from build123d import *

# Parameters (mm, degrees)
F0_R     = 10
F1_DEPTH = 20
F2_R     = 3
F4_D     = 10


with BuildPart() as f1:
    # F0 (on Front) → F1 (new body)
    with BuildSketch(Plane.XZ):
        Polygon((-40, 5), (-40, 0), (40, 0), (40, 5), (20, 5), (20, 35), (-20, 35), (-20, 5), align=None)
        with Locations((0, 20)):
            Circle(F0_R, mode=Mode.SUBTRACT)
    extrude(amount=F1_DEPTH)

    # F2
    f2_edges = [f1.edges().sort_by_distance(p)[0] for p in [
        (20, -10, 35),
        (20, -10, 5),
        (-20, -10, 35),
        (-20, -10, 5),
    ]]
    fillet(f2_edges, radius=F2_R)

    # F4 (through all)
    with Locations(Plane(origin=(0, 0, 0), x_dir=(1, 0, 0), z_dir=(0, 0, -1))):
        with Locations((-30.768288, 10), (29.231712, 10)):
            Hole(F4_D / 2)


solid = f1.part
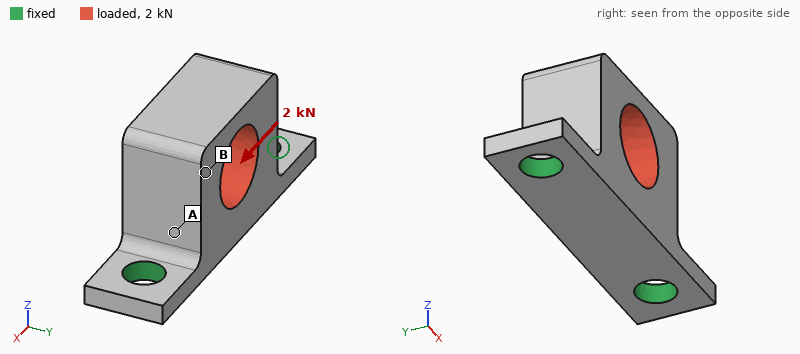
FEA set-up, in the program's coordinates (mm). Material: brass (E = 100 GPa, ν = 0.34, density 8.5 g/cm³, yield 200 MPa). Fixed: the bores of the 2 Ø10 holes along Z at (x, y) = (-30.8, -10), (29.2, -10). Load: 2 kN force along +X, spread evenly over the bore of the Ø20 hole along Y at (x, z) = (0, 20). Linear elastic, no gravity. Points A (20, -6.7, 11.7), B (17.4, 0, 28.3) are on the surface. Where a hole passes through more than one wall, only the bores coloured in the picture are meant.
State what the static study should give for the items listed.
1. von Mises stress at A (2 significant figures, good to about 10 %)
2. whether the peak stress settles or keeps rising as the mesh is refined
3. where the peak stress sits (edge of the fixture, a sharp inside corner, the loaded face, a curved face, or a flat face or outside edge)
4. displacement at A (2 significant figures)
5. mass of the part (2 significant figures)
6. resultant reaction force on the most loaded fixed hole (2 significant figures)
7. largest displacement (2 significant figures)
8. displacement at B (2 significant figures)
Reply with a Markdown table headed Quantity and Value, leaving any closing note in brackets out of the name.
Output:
| Quantity | Value |
|---|---|
| von Mises stress at A | 9.5 MPa |
| whether the peak stress settles or keeps rising as the mesh is refined | keeps rising |
| where the peak stress sits | edge of the fixture |
| displacement at A | 3.7 µm |
| mass of the part | 210 g |
| resultant reaction force on the most loaded fixed hole | 1.3 kN |
| largest displacement | 11 µm |
| displacement at B | 8.6 µm |
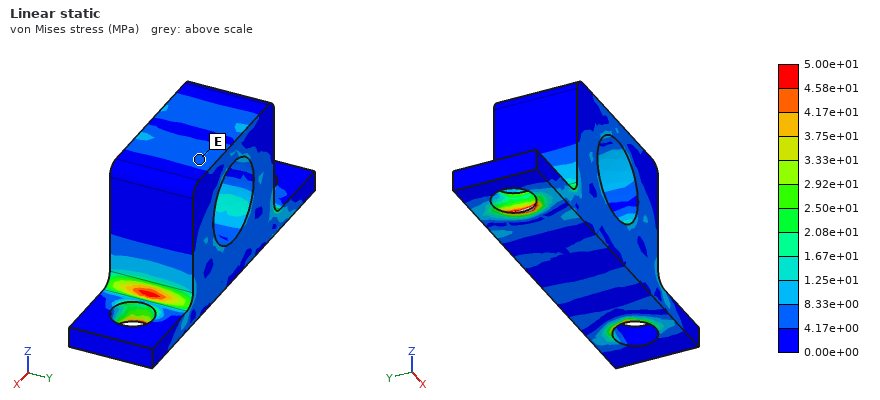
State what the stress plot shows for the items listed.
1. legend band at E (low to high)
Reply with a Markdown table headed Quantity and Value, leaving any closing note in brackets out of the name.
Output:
| Quantity | Value |
|---|---|
| legend band at E | 4.17e+00 to 8.33e+00 MPa |
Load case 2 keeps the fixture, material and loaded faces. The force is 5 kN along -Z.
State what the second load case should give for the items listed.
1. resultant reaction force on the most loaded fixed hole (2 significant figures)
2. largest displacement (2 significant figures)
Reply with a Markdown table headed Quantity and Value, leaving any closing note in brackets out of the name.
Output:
| Quantity | Value |
|---|---|
| resultant reaction force on the most loaded fixed hole | 3.0 kN |
| largest displacement | 18 µm |
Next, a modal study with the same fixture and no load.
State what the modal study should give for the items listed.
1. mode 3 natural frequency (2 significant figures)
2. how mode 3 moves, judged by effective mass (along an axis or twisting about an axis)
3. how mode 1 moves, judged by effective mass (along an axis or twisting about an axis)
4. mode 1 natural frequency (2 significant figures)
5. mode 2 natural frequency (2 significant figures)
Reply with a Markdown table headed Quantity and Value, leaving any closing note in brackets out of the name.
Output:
| Quantity | Value |
|---|---|
| mode 3 natural frequency | 6900 Hz |
| how mode 3 moves, judged by effective mass | along Z |
| how mode 1 moves, judged by effective mass | along Y |
| mode 1 natural frequency | 2200 Hz |
| mode 2 natural frequency | 6200 Hz |
